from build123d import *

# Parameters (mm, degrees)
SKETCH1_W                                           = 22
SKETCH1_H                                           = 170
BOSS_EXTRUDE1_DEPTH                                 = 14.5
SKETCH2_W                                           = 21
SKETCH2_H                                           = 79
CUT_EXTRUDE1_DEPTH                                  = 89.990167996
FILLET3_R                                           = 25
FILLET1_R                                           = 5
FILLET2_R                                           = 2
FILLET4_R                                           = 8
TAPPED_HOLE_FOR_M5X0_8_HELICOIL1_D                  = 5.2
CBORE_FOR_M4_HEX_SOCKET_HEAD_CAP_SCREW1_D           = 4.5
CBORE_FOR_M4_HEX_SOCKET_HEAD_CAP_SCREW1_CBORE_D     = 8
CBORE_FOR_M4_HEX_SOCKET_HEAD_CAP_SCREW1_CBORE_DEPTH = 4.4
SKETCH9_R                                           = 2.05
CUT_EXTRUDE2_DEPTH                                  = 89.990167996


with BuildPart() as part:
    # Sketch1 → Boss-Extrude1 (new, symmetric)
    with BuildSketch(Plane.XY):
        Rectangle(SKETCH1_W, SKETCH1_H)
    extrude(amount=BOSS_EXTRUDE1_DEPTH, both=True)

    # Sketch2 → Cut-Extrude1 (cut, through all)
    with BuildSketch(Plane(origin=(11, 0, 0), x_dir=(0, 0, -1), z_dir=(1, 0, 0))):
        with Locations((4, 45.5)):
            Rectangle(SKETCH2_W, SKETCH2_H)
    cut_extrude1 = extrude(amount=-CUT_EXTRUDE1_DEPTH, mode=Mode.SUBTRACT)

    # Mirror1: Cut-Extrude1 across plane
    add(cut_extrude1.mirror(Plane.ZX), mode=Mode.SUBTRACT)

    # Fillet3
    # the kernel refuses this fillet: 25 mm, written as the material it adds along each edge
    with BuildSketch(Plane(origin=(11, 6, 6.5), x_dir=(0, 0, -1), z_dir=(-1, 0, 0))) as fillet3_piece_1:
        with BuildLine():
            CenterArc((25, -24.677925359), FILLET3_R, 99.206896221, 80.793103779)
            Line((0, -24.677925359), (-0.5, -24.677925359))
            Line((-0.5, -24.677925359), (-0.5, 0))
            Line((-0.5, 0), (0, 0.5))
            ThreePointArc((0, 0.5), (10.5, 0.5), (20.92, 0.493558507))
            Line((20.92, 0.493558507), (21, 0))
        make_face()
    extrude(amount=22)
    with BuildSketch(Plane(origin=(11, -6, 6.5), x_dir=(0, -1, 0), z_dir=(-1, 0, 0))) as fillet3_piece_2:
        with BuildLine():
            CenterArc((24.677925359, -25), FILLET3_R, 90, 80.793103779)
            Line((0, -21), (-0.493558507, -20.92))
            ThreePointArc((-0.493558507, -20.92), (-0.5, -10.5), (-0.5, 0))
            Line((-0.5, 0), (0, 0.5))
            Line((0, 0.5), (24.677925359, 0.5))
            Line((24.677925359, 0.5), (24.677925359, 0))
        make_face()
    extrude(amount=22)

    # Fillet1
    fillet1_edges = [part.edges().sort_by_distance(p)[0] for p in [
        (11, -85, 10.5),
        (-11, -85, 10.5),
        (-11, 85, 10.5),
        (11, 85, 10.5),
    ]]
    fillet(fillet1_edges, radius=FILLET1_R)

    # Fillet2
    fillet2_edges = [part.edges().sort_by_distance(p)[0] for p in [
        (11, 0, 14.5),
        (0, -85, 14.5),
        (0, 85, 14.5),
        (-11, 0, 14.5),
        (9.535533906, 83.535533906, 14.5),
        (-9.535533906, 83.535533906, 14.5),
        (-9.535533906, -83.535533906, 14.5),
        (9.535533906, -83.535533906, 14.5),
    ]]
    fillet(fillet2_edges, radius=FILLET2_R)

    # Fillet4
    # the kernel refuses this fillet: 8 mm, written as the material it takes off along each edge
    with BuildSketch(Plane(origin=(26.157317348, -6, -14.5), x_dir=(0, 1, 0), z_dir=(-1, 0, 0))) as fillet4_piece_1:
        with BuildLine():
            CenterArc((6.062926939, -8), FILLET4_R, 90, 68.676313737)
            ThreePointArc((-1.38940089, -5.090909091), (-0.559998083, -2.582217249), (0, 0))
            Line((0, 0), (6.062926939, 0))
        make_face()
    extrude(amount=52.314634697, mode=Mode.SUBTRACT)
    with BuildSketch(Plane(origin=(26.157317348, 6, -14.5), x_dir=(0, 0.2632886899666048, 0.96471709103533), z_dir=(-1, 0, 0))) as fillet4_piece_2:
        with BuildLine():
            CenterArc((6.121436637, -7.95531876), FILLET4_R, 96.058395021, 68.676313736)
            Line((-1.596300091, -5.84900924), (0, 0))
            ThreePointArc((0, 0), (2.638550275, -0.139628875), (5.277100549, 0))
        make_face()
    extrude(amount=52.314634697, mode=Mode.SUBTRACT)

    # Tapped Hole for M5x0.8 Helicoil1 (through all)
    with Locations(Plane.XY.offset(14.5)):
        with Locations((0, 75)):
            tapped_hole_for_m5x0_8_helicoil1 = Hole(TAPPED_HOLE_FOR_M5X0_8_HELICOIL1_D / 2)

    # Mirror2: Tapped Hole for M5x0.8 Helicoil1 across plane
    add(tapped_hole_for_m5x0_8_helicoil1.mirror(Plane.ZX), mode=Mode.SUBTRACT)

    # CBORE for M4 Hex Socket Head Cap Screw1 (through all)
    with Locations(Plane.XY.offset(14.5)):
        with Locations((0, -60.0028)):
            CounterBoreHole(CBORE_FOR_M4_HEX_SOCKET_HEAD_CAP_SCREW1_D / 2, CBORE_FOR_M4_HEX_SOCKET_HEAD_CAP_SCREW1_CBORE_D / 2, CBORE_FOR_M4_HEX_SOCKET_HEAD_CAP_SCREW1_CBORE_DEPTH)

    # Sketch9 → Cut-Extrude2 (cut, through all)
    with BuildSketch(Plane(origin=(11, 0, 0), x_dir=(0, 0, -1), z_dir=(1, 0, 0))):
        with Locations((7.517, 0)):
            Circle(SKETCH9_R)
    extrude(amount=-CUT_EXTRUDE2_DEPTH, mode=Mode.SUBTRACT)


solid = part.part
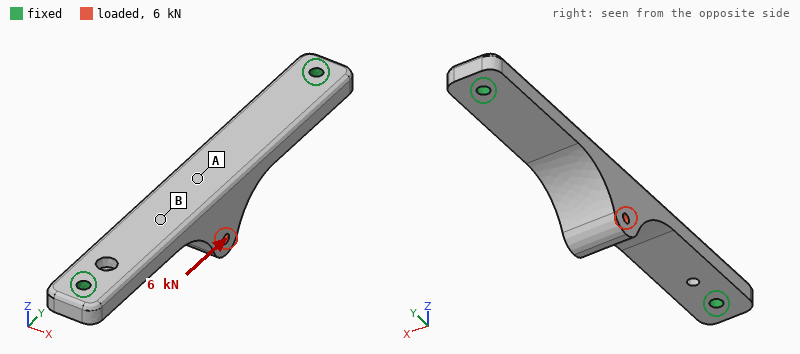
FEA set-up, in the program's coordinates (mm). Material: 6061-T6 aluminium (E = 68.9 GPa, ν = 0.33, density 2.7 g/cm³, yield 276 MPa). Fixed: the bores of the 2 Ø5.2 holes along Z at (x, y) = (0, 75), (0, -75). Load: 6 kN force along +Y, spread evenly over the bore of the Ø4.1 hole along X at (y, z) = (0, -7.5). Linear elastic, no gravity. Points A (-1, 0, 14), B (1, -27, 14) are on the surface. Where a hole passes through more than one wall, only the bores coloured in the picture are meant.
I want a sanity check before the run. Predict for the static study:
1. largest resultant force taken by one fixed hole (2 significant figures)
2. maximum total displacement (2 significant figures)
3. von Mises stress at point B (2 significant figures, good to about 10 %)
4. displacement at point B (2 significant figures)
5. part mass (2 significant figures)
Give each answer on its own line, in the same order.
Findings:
3.3 kN
0.16 mm
84 MPa
0.13 mm
110 g
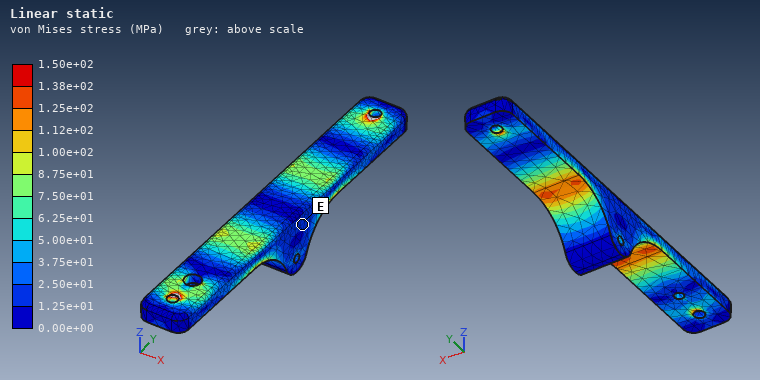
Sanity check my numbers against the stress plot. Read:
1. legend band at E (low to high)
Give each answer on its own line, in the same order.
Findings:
1.25e+01 to 2.50e+01 MPa
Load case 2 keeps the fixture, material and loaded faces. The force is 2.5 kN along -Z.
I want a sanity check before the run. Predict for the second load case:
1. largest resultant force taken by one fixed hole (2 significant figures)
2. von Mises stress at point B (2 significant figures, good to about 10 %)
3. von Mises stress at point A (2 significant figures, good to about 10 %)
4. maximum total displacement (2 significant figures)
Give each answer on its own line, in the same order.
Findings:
1.7 kN
87 MPa
33 MPa
0.35 mm
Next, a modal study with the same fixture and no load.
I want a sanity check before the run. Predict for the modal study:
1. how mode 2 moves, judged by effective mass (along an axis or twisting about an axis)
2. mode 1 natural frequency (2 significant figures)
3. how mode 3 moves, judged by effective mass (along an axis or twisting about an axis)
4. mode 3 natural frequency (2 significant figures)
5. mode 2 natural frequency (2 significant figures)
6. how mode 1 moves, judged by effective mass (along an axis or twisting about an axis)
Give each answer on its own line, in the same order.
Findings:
along X
1700 Hz
along X
4000 Hz
2300 Hz
along Z
